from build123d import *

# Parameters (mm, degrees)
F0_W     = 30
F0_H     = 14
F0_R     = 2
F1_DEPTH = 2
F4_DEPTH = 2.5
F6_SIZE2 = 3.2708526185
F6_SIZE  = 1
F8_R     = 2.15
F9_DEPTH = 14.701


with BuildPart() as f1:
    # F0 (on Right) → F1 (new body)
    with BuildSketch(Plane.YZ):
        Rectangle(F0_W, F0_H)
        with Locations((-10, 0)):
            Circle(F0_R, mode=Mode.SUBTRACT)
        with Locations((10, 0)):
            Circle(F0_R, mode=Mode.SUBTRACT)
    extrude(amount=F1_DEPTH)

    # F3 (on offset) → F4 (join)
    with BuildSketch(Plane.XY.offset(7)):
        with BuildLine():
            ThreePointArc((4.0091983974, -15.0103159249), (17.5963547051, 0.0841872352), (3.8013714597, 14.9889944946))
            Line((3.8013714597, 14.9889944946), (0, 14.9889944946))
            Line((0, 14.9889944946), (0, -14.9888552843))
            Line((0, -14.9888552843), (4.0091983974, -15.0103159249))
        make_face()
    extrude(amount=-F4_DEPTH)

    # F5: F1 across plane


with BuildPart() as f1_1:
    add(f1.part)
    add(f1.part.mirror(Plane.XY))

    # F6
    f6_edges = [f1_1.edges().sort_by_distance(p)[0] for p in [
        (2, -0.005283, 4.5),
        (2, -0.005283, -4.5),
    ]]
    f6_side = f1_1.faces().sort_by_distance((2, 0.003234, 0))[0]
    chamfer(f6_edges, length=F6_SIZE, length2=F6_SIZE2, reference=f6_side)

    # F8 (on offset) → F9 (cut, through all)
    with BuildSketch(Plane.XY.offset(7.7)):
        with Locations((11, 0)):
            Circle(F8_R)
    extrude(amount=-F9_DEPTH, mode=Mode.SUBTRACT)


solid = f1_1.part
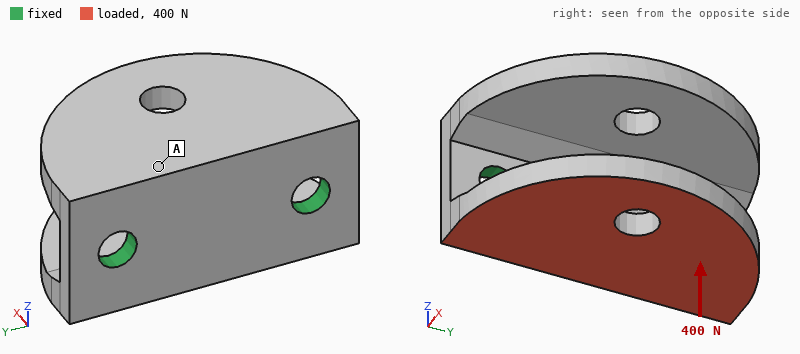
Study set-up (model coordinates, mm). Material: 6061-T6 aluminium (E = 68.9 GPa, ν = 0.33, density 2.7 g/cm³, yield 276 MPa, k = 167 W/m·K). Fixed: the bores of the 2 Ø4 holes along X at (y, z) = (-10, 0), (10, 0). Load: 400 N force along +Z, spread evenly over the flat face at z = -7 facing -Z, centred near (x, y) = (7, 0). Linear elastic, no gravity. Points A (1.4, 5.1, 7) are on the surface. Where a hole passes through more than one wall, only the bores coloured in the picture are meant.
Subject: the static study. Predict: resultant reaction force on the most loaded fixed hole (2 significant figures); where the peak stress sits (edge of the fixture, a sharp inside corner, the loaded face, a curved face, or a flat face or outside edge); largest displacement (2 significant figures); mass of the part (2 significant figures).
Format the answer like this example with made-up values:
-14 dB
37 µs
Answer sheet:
200 N
a flat face or outside edge
0.15 mm
7.2 g
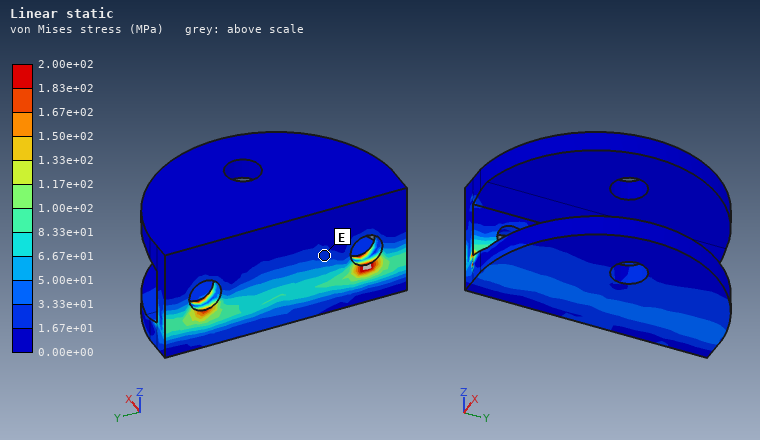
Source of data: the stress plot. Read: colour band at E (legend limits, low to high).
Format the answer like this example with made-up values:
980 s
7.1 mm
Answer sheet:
1.67e+01 to 3.33e+01 MPa
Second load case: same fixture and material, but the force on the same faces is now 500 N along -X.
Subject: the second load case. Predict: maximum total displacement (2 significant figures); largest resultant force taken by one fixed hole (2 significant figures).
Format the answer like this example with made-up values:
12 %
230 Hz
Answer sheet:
0.11 mm
250 N
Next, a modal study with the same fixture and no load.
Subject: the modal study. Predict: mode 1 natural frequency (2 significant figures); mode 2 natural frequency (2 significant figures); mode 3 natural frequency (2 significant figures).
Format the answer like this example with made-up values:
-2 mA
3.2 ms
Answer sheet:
6200 Hz
6400 Hz
14 kHz
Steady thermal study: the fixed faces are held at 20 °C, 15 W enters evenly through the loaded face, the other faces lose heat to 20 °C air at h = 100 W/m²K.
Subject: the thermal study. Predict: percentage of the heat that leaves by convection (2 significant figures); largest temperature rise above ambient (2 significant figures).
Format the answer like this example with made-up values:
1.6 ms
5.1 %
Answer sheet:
6.1 %
15 K
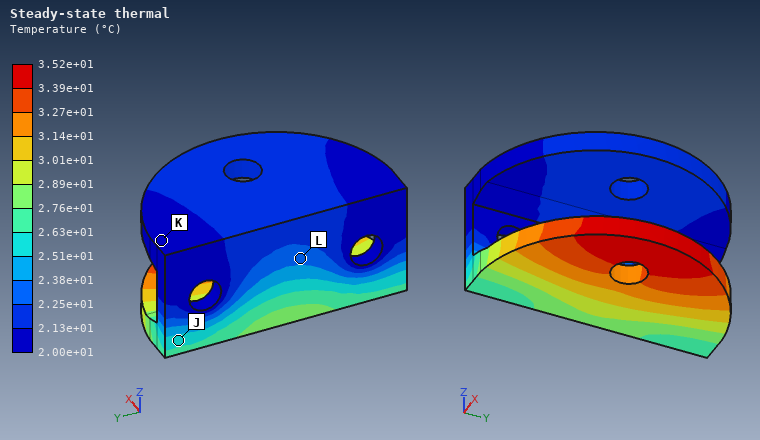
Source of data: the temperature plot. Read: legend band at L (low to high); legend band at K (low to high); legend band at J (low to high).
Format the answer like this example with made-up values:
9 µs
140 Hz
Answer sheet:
2.25e+01 to 2.38e+01 °C
2.00e+01 to 2.13e+01 °C
2.51e+01 to 2.63e+01 °C
